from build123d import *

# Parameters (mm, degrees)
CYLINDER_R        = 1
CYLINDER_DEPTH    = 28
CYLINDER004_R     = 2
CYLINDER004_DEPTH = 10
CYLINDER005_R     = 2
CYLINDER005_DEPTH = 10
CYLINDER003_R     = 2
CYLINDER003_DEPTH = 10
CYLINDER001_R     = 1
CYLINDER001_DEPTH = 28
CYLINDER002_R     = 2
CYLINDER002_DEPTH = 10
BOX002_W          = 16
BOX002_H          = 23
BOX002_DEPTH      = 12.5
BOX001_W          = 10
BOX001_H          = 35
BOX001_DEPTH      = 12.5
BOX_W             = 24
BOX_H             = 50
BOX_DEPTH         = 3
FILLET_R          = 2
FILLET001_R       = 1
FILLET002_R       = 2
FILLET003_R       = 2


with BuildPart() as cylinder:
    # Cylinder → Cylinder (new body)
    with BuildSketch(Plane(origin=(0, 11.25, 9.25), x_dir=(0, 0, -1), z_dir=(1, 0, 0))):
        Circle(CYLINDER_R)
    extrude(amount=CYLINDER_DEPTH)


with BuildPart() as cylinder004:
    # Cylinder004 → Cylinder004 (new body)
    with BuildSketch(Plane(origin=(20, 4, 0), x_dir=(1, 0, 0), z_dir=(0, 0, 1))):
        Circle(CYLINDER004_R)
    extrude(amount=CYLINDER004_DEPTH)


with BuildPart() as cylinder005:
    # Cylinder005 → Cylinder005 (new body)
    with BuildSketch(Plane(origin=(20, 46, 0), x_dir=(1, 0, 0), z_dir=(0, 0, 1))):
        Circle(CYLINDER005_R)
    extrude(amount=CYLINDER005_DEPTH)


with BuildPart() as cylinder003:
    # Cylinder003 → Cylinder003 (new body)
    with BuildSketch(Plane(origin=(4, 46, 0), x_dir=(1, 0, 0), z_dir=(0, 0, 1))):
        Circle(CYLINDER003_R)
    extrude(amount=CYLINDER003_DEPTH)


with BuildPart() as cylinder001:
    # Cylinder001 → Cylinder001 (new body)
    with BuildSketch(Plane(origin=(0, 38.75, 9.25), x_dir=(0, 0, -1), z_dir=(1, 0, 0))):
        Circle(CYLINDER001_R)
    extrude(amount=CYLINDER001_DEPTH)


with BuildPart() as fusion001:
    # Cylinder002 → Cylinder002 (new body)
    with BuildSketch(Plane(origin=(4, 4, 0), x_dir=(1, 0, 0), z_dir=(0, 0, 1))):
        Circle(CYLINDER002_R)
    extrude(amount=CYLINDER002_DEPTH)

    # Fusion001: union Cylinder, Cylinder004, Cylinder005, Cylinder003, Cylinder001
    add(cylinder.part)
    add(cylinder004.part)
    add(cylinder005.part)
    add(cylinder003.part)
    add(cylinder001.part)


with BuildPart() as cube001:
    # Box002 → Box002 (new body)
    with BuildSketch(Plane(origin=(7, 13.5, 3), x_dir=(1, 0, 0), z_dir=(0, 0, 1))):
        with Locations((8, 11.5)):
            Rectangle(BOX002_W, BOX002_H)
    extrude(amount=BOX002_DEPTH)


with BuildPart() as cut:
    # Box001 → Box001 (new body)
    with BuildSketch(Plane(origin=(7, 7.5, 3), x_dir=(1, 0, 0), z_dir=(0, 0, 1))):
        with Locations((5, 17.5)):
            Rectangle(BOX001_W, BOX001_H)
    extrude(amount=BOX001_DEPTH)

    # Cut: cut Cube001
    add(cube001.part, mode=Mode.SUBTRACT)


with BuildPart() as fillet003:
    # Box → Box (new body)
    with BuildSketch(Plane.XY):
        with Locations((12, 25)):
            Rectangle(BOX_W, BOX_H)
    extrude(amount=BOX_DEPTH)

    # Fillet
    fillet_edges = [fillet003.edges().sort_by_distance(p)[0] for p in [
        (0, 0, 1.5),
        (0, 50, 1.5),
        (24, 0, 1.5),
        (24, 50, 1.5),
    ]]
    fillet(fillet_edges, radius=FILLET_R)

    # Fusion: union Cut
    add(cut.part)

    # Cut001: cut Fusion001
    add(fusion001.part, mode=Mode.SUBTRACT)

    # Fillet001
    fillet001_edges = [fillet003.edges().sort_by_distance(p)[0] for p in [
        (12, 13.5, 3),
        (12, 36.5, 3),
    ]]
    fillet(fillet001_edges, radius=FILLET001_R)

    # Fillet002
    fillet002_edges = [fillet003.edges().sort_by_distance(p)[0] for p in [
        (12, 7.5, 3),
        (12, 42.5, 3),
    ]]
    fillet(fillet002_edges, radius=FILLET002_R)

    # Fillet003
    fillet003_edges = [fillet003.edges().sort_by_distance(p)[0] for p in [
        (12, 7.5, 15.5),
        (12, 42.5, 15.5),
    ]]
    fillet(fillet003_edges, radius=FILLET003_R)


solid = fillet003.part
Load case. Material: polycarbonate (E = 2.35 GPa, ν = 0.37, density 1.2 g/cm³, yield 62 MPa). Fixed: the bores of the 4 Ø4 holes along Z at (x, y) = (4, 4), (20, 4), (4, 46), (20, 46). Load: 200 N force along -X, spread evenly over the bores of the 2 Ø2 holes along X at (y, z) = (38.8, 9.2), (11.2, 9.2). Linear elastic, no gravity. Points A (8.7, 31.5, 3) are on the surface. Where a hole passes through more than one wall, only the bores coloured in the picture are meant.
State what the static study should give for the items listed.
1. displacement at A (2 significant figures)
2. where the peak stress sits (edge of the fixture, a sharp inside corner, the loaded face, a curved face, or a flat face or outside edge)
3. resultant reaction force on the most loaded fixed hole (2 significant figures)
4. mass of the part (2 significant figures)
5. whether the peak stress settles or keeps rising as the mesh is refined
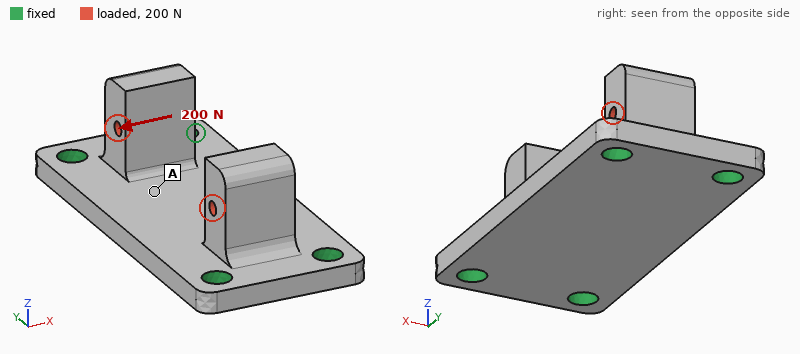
0.025 mm
a sharp inside corner
84 N
5.9 g
keeps rising
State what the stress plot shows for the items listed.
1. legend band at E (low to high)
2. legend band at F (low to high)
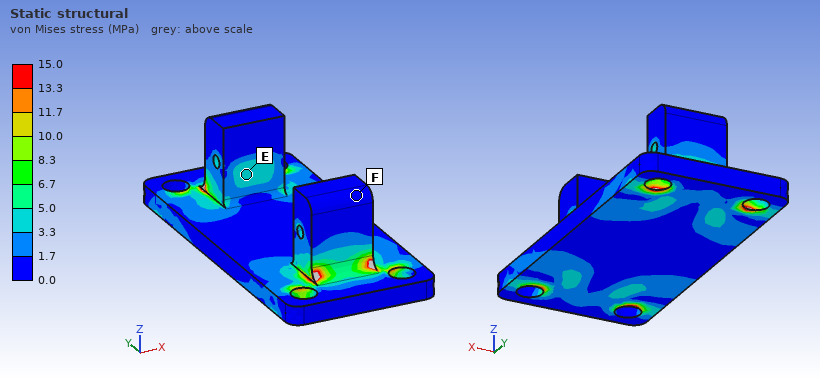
3.3 to 5.0 MPa
0.0 to 1.7 MPa
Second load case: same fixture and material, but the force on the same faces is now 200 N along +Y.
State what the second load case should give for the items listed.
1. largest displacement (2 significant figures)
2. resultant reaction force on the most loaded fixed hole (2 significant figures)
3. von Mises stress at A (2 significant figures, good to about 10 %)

0.20 mm
55 N
4.9 MPa
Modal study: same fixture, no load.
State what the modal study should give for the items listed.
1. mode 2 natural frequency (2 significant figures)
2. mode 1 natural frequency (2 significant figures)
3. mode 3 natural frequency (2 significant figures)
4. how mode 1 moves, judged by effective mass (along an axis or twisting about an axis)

4000 Hz
2200 Hz
4100 Hz
along Z
